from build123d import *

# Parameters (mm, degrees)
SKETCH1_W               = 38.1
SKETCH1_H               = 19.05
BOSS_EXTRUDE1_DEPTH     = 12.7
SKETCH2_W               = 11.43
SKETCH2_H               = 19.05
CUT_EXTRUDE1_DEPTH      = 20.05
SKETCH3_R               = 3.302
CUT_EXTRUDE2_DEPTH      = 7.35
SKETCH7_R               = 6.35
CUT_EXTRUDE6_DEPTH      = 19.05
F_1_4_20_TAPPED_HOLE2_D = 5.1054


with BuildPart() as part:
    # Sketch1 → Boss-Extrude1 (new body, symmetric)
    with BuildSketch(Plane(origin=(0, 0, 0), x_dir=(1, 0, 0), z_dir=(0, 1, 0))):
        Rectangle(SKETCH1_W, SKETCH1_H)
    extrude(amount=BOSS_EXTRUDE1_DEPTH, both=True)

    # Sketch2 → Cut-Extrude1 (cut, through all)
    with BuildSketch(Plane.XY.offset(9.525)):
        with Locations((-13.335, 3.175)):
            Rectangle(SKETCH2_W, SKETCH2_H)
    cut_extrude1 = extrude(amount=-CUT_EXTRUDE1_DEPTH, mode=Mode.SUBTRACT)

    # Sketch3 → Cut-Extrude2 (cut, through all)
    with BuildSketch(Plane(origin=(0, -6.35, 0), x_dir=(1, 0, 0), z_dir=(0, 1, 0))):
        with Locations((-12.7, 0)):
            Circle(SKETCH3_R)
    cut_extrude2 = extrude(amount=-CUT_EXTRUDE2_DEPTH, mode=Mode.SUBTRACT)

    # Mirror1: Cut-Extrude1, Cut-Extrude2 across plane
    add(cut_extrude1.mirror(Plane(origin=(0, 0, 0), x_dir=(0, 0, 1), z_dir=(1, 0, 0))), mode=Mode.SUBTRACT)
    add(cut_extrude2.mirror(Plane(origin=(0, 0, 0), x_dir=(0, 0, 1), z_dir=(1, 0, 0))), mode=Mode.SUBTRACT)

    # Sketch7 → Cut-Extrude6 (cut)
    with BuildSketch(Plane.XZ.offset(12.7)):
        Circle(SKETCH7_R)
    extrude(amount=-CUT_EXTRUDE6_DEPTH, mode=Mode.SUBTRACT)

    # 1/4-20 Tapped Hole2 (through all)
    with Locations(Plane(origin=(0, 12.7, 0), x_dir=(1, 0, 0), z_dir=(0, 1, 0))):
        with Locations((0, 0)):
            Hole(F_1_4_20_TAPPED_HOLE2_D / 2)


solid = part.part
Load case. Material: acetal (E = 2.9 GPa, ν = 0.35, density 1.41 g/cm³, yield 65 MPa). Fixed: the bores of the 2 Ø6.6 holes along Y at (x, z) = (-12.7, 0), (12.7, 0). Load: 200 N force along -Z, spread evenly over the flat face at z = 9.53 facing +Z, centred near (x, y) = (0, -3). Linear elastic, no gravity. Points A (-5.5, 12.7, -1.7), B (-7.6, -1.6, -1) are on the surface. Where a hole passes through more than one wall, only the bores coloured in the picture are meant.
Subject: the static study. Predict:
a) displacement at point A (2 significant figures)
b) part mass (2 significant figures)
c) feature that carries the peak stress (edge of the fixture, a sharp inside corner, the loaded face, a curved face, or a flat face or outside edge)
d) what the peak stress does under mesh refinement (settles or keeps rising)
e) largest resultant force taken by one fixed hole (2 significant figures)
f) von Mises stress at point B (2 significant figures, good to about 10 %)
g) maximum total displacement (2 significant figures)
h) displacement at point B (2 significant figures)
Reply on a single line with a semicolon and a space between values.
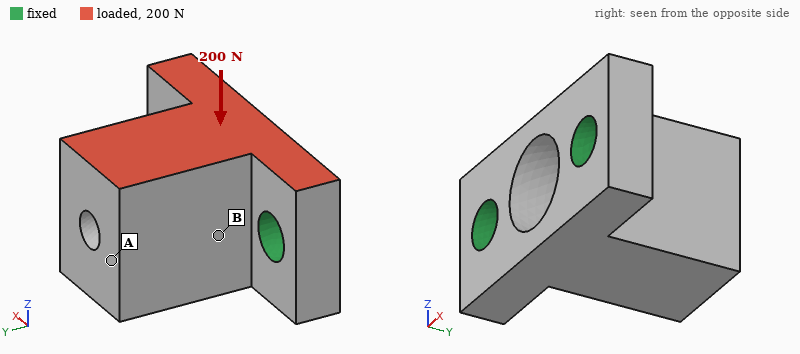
70 µm; 10 g; edge of the fixture; keeps rising; 100 N; 2.9 MPa; 76 µm; 27 µm
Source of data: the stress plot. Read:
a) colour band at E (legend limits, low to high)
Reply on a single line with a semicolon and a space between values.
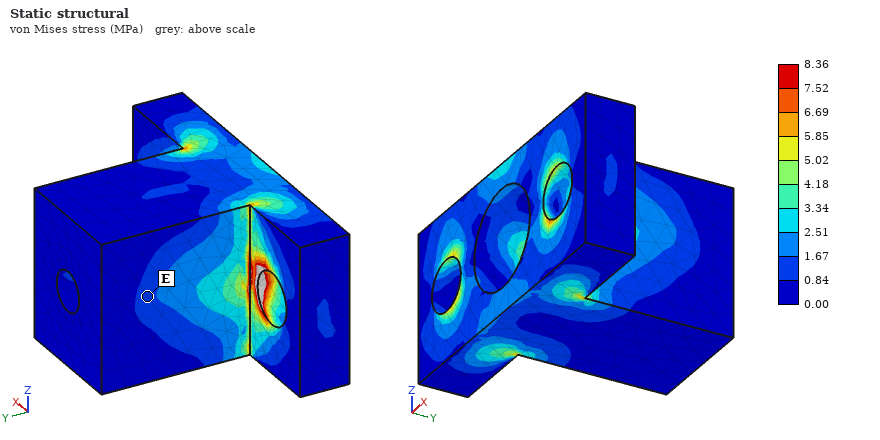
0.84 to 1.67 MPa
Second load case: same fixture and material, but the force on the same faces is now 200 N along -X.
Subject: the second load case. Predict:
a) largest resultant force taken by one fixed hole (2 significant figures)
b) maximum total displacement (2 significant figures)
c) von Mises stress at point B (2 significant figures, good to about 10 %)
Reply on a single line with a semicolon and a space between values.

130 N; 49 µm; 2.0 MPa
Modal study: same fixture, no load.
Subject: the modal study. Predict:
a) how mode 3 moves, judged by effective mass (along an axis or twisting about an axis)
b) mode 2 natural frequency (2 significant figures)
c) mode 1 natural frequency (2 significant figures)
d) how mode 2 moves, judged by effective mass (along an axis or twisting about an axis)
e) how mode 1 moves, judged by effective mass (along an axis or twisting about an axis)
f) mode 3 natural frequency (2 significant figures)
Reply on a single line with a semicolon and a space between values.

along Y; 4200 Hz; 2800 Hz; along X; along Z; 7800 Hz
